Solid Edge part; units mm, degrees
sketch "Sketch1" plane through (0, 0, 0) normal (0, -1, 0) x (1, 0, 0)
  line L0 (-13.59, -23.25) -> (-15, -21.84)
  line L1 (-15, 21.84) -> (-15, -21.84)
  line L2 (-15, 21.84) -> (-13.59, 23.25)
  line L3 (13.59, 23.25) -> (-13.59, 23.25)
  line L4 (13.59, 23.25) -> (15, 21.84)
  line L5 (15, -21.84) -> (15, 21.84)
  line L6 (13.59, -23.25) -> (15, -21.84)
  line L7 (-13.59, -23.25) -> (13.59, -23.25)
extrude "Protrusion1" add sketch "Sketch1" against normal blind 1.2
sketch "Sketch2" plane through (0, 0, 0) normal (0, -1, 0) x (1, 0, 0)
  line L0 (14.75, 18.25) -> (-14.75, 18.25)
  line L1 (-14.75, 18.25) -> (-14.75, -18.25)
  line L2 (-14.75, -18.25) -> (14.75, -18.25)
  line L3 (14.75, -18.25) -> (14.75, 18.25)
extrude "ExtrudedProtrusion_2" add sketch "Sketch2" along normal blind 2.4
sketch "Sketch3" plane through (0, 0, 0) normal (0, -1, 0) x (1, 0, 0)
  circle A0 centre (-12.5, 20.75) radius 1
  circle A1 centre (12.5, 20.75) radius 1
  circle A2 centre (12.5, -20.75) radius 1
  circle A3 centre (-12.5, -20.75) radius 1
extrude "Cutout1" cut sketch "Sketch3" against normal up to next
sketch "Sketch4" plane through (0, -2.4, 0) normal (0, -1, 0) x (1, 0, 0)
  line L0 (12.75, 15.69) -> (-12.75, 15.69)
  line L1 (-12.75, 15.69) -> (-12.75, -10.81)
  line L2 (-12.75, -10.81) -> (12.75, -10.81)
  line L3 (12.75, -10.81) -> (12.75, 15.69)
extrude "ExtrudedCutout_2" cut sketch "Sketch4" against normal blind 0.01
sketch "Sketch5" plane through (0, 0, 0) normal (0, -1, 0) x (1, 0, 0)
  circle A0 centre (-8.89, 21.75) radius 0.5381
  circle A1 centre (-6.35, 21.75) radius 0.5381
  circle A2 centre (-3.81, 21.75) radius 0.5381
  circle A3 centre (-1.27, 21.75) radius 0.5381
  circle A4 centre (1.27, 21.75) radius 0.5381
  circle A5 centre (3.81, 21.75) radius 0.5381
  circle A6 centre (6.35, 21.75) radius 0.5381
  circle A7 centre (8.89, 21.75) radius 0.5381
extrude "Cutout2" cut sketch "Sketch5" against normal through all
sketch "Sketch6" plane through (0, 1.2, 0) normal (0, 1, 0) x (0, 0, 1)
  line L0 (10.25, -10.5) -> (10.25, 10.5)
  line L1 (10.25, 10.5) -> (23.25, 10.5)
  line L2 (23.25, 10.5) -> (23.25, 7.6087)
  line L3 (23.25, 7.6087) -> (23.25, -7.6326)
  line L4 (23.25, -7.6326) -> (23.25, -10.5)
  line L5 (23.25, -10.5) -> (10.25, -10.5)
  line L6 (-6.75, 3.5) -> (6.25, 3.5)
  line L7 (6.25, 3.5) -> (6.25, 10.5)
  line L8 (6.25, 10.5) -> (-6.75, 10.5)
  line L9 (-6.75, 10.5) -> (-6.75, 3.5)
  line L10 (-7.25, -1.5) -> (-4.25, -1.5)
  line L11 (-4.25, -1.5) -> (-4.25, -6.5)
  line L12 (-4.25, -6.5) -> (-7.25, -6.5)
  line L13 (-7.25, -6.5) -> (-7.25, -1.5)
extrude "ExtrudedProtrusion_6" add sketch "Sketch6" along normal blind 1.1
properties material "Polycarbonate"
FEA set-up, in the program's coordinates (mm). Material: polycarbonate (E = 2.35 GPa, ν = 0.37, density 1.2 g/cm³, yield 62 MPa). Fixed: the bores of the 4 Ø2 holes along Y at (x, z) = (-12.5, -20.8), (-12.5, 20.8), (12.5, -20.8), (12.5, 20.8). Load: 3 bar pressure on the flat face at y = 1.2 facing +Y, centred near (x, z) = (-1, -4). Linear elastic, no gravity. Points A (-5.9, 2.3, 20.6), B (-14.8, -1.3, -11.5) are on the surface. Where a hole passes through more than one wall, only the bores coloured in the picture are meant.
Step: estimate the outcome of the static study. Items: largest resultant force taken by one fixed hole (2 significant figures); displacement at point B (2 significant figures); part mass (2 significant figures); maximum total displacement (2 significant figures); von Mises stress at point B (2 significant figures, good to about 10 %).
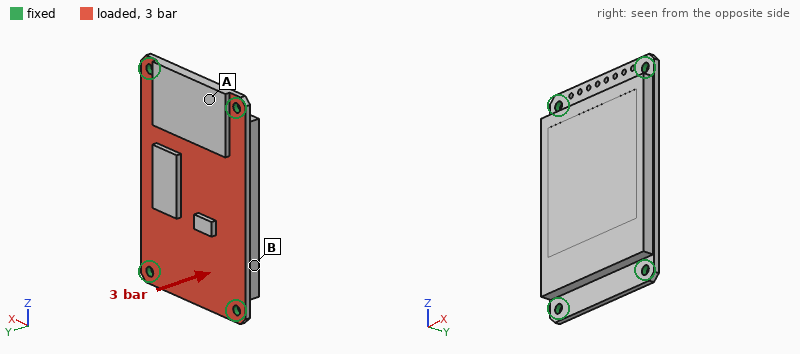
160 N
0.37 mm
5.6 g
0.60 mm
11 MPa
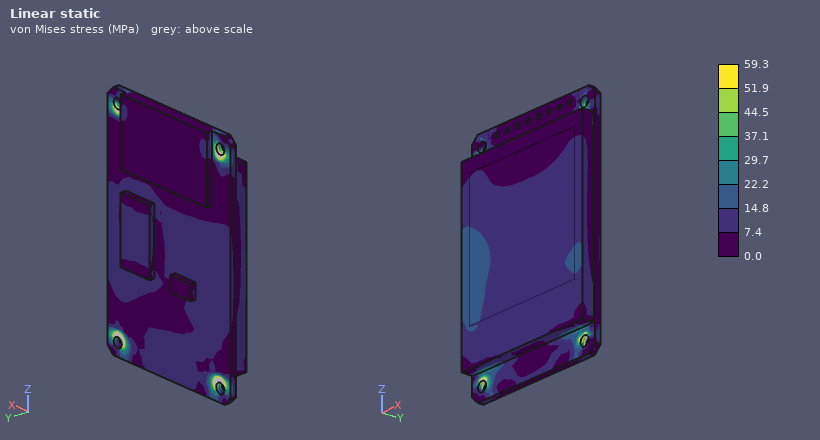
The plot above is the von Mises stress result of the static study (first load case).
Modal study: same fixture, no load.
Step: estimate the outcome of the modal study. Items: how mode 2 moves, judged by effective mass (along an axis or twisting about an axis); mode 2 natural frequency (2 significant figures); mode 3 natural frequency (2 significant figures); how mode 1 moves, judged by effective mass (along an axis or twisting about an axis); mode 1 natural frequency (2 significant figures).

twisting about Z
3000 Hz
4100 Hz
along Y
1800 Hz
